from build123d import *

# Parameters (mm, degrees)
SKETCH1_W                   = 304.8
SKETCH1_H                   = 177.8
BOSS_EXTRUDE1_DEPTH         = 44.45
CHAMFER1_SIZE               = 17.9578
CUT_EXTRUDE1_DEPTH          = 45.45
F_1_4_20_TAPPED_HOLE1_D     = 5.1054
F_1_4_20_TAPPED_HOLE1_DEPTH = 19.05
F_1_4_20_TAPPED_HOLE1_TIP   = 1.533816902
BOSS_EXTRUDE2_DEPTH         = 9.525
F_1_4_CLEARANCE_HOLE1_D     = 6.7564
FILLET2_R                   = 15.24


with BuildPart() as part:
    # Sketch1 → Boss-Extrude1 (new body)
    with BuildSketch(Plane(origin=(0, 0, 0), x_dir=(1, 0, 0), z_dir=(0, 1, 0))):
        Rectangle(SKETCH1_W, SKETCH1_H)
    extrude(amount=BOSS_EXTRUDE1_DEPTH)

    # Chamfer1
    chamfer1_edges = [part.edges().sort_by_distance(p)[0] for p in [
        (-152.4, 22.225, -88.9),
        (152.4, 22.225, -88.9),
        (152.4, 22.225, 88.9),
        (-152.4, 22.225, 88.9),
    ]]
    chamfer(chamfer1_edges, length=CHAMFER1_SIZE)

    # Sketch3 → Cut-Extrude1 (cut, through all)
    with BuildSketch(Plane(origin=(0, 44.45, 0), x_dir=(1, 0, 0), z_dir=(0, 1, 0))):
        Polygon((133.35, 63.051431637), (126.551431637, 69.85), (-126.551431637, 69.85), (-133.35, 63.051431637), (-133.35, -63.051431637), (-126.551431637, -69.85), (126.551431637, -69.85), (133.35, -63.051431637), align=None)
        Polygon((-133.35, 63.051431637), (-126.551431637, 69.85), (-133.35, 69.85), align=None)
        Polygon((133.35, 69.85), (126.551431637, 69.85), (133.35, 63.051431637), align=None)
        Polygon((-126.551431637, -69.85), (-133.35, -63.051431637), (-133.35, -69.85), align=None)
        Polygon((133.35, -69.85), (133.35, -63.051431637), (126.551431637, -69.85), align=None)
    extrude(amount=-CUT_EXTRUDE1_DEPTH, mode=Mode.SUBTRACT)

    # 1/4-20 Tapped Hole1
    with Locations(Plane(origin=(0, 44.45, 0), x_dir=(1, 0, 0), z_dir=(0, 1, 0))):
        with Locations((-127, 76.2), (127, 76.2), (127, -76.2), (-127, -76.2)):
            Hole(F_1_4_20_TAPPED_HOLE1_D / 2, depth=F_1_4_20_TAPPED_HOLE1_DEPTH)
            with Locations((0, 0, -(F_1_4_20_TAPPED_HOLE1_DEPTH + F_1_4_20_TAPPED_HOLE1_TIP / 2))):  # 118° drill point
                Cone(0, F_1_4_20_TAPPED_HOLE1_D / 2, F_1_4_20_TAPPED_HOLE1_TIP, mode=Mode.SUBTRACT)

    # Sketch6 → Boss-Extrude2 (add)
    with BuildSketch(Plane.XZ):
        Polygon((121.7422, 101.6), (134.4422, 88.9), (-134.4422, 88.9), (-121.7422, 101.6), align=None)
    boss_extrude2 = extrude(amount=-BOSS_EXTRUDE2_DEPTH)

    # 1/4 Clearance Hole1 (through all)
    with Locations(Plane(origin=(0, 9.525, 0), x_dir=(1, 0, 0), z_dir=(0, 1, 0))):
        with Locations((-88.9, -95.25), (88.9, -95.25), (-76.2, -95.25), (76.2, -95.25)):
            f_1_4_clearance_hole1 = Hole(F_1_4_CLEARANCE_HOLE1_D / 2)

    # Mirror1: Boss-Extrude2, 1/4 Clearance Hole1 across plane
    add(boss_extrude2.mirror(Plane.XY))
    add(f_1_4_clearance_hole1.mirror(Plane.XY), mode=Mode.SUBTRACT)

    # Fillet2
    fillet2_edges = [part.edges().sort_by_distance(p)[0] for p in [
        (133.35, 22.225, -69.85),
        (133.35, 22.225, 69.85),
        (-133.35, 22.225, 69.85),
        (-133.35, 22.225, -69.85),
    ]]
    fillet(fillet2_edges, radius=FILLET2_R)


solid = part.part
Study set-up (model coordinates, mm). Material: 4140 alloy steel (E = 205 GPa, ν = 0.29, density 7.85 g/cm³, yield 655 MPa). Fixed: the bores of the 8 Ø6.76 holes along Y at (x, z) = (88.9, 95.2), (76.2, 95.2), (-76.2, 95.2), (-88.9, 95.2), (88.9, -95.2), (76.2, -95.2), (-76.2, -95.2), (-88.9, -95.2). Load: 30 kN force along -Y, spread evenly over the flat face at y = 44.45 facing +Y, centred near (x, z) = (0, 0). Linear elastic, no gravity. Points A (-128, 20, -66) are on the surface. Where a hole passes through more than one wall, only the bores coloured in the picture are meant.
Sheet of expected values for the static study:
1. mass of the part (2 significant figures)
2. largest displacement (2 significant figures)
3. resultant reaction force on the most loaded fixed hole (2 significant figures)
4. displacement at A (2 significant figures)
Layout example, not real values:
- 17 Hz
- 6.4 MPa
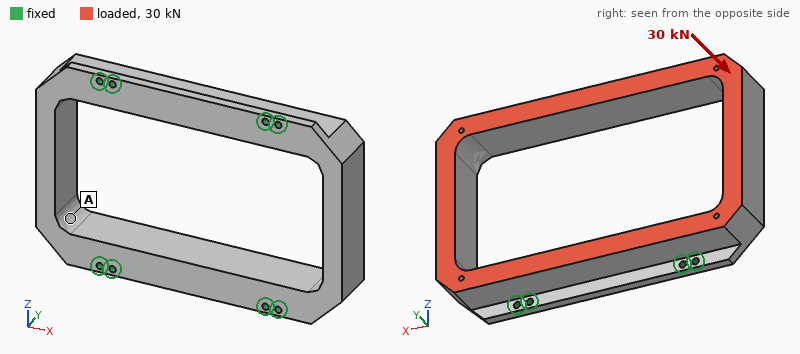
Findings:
- 6.2 kg
- 46 µm
- 6.2 kN
- 24 µm
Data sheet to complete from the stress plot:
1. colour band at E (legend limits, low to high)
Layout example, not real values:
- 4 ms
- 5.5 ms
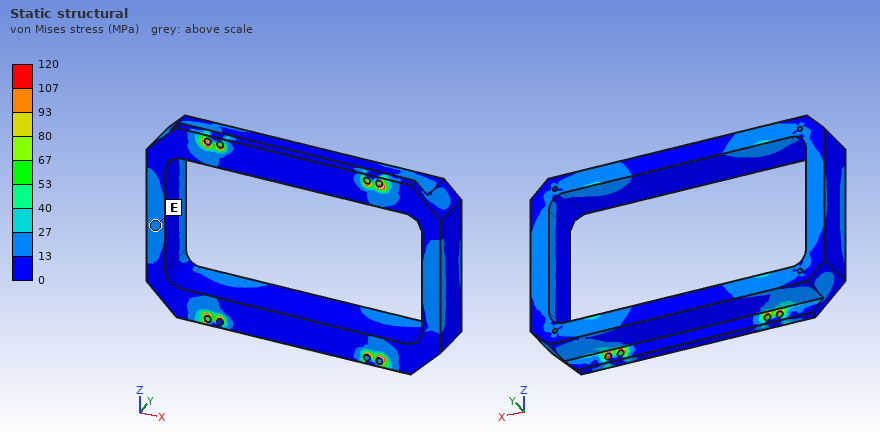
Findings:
- 13 to 27 MPa
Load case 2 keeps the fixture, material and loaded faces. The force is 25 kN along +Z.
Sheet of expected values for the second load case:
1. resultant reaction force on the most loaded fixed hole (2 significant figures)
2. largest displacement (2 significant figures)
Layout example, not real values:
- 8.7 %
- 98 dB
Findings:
- 6.4 kN
- 56 µm
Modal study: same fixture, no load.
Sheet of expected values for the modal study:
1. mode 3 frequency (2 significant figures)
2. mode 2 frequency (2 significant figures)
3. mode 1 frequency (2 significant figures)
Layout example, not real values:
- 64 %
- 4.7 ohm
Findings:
- 2300 Hz
- 1900 Hz
- 1900 Hz
